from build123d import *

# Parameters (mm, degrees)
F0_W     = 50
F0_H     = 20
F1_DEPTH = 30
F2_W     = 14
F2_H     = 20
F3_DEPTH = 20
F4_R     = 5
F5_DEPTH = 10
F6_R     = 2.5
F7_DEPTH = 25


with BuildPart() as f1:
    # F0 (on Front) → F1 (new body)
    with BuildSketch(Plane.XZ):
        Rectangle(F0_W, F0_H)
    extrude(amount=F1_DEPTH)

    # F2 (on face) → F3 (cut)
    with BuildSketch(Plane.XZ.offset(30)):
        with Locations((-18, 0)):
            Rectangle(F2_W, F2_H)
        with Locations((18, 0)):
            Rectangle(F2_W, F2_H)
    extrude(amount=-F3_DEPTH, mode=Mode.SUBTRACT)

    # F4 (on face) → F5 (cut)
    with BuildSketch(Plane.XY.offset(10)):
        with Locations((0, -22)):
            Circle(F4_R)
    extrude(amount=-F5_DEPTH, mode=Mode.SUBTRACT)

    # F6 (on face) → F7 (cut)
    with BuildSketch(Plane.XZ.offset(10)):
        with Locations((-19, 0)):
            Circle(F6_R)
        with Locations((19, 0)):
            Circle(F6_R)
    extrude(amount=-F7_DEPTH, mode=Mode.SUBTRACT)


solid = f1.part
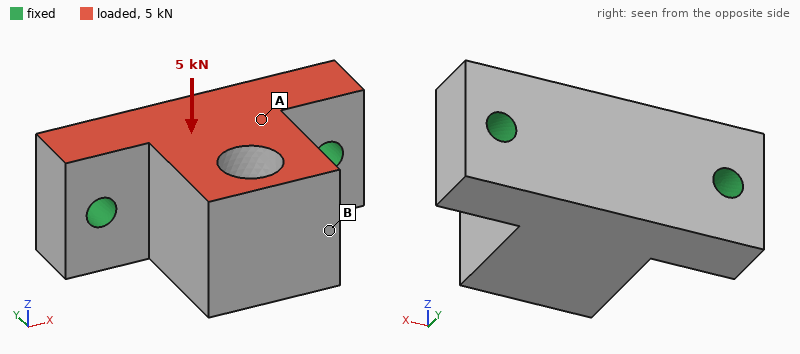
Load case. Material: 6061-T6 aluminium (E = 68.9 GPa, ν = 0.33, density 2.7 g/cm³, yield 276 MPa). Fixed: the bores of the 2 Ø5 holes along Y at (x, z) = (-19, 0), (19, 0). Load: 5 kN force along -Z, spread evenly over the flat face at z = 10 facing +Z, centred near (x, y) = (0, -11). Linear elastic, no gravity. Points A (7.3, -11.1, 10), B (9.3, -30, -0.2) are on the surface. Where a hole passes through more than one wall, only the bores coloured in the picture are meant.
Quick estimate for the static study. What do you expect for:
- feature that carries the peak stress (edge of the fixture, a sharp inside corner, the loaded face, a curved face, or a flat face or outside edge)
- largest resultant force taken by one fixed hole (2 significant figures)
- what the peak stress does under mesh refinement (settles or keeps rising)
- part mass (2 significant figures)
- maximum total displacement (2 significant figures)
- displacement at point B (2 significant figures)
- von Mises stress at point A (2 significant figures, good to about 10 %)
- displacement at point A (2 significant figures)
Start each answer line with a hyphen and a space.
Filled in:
- edge of the fixture
- 2.5 kN
- keeps rising
- 48 g
- 49 µm
- 46 µm
- 19 MPa
- 21 µm
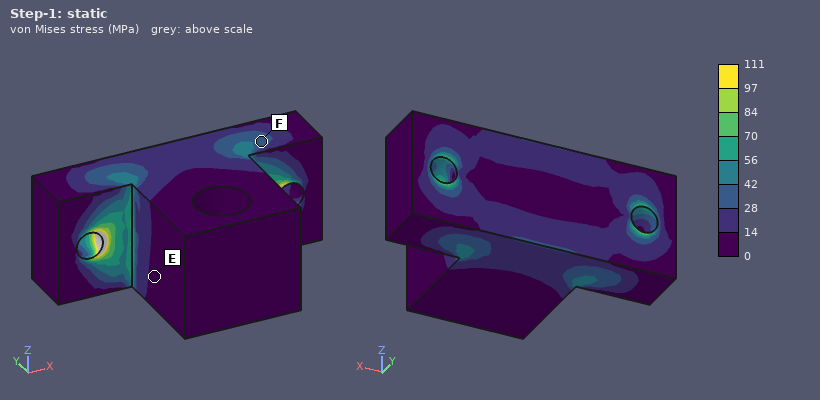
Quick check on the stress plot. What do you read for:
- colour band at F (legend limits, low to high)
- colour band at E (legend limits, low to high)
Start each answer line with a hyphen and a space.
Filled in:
- 28 to 42 MPa
- 0 to 14 MPa
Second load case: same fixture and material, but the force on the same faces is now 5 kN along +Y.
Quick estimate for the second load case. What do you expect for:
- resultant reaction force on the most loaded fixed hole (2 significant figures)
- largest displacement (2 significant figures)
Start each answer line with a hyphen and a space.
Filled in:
- 2.5 kN
- 57 µm
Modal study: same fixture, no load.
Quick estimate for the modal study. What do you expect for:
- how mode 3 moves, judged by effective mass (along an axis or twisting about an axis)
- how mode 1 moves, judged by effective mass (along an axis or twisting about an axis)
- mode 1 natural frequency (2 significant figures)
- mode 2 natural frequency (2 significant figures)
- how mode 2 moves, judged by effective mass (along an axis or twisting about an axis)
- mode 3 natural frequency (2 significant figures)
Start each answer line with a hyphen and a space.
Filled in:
- along Y
- along Z
- 8300 Hz
- 16 kHz
- along X
- 18 kHz
